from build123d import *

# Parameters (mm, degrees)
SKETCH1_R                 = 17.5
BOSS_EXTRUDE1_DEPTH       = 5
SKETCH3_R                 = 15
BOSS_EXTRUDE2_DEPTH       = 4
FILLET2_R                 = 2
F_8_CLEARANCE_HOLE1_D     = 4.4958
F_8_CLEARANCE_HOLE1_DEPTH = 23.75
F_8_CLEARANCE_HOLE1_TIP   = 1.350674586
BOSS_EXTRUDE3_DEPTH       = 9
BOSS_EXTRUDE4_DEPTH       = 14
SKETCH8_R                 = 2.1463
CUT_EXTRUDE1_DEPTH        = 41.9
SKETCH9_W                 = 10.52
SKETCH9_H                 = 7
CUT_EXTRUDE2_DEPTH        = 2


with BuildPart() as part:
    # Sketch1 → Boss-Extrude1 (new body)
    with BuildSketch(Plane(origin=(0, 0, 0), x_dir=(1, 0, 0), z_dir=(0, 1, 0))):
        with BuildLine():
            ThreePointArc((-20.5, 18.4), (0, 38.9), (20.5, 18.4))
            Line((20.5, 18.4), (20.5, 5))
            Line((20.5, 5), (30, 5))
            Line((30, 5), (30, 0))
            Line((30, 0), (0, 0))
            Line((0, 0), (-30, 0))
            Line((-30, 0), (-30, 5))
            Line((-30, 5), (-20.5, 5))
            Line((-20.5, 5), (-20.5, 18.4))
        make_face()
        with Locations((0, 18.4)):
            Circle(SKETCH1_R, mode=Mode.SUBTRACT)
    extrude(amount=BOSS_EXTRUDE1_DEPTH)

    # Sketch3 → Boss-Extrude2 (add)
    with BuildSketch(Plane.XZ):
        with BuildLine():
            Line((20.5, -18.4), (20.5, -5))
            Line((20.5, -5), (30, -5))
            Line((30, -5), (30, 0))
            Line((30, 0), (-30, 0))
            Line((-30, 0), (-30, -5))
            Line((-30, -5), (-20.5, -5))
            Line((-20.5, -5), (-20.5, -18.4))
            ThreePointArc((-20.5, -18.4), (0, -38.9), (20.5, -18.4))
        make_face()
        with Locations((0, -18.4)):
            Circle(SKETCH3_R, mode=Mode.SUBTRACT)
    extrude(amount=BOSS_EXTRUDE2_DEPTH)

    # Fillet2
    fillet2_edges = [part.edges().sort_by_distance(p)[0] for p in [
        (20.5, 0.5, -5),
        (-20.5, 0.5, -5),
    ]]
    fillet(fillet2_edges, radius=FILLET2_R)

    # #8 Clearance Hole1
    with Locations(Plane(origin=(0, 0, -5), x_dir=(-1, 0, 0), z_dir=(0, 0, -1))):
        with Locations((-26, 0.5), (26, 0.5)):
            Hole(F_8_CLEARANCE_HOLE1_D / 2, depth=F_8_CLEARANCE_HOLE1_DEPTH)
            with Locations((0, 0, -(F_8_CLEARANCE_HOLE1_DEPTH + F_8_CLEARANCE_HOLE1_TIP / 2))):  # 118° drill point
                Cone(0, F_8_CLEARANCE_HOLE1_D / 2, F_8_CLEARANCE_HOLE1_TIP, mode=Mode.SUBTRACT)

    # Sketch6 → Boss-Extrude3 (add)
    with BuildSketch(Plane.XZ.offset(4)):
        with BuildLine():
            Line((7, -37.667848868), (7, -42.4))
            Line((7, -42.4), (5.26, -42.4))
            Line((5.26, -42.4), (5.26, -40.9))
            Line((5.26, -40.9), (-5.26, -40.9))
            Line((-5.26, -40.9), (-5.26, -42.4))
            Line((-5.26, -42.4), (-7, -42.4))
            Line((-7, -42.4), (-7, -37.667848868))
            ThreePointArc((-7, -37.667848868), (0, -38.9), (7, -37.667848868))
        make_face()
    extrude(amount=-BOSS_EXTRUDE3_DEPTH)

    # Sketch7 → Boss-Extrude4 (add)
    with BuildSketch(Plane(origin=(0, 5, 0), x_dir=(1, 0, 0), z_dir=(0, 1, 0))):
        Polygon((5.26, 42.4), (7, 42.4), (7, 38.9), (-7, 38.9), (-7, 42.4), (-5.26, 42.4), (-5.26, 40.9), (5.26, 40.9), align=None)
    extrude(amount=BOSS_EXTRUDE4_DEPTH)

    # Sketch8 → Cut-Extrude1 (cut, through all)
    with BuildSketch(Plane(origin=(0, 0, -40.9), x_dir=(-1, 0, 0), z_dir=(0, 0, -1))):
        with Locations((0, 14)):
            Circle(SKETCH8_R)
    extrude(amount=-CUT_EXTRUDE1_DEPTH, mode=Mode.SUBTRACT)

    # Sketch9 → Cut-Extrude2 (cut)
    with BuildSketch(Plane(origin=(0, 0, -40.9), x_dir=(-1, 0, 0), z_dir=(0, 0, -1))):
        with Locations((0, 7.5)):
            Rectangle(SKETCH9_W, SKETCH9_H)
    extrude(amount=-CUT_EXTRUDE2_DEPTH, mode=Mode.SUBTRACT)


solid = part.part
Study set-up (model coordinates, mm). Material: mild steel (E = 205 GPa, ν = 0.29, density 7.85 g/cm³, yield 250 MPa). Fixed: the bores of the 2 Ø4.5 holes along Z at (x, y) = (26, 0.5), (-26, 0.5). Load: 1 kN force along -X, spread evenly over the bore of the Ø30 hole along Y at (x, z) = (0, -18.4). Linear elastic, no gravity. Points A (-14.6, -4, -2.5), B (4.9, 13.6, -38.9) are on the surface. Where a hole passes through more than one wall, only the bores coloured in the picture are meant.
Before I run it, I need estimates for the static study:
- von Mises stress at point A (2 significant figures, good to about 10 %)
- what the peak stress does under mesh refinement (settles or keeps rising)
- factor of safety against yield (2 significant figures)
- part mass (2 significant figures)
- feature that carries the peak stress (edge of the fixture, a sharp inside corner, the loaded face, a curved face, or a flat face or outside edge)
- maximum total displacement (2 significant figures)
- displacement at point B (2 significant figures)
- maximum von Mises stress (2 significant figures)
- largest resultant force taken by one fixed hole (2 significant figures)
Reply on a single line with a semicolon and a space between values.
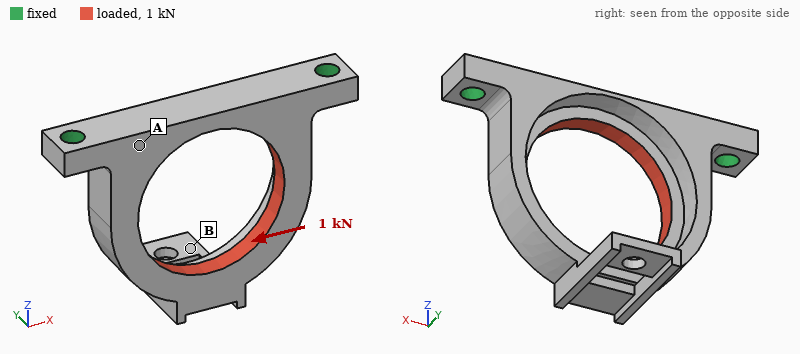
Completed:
21 MPa; settles; 3.0; 51 g; a curved face; 28 µm; 26 µm; 84 MPa; 580 N
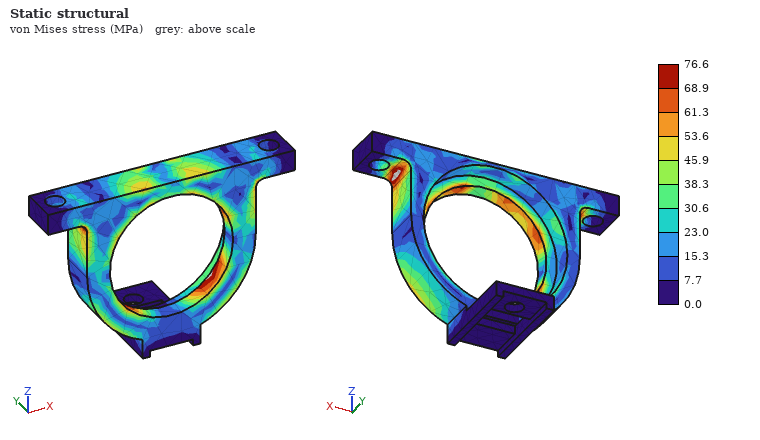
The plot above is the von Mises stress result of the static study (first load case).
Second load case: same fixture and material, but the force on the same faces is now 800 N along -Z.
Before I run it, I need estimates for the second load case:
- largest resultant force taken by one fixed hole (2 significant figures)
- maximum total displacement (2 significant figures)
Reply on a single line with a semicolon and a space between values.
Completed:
400 N; 19 µm
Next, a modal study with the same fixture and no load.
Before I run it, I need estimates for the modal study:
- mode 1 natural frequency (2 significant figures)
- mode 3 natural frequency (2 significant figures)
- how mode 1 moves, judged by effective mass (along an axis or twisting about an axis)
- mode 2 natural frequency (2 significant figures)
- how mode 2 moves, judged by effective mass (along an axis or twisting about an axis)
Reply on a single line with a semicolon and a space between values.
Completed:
2300 Hz; 6100 Hz; along Y; 4600 Hz; along X
